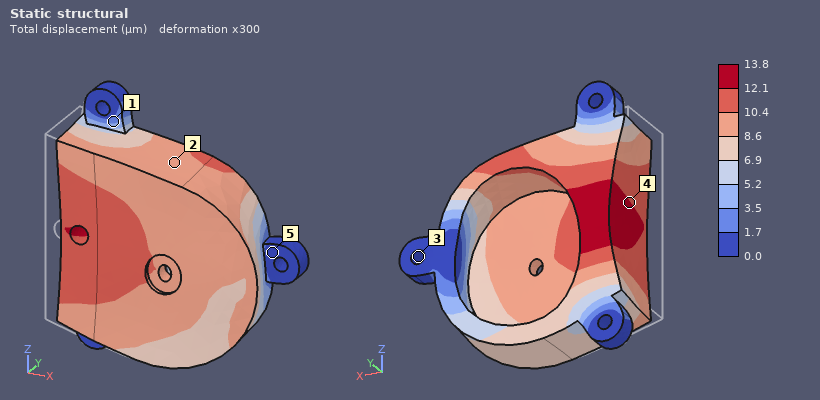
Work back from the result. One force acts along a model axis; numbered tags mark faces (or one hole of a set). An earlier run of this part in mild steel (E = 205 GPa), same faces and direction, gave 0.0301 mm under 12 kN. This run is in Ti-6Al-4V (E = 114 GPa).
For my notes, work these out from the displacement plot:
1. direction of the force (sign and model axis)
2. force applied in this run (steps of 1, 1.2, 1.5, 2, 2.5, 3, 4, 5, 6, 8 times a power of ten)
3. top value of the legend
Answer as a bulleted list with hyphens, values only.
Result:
- +X
- 3 kN
- 13.8 µm
